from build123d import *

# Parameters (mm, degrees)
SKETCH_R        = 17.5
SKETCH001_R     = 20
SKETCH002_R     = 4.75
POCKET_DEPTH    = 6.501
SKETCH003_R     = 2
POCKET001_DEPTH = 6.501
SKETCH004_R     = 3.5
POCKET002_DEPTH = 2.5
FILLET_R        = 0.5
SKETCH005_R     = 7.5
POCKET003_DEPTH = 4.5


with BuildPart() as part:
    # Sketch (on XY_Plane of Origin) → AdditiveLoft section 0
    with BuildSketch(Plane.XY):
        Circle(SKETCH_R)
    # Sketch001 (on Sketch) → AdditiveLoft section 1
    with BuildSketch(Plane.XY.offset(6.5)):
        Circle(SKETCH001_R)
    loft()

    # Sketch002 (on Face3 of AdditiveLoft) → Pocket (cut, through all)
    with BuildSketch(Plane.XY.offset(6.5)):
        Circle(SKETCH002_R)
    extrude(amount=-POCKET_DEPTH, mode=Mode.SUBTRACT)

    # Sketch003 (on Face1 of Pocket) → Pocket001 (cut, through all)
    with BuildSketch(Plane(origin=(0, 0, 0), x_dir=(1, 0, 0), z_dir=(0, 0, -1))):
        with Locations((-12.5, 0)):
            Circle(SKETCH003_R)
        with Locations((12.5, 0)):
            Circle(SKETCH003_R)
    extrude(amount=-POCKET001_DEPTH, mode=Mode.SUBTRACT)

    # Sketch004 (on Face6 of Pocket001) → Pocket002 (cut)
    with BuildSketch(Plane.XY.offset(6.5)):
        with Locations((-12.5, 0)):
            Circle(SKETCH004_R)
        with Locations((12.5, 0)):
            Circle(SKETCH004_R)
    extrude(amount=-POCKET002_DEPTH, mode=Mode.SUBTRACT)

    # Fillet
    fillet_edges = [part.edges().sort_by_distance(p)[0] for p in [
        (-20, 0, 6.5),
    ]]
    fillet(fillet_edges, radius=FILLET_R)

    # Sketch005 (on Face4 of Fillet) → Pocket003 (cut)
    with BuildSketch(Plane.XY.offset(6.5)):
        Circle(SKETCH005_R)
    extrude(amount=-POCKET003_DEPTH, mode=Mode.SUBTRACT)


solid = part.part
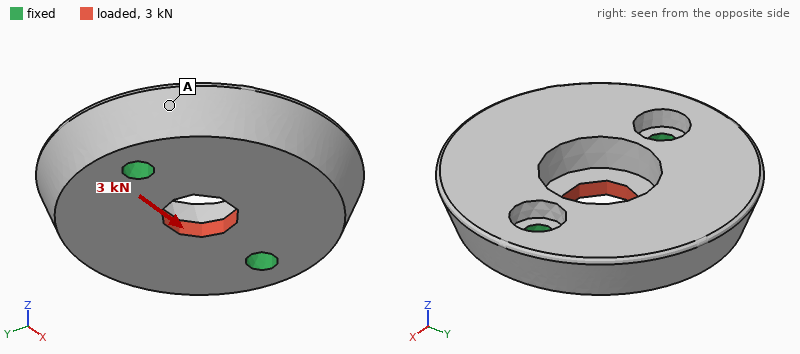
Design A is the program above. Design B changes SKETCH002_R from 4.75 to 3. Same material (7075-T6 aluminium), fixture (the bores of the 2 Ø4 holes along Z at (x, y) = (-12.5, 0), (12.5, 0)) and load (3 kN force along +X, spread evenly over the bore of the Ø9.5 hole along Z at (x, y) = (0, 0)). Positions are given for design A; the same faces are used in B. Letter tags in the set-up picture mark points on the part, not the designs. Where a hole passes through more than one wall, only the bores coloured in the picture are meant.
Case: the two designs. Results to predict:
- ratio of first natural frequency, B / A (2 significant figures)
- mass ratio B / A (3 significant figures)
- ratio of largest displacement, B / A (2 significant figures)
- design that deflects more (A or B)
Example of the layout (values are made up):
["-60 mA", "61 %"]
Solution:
["1.00", "1.01", "1.3", "B"]
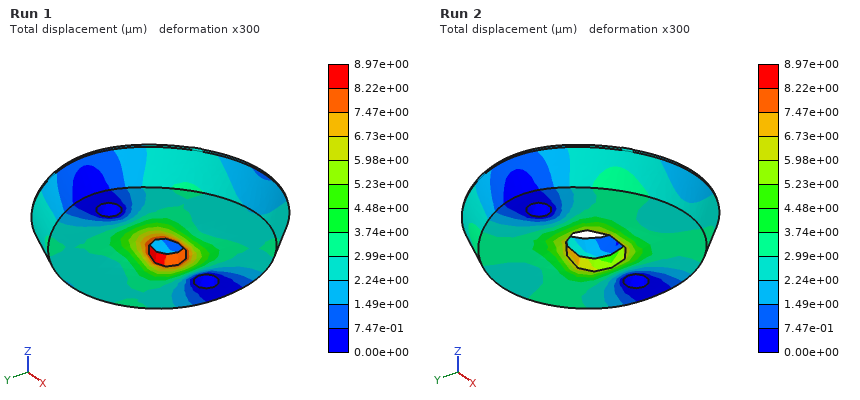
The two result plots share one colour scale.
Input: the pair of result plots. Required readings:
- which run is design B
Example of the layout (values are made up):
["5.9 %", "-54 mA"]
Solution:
["Run 1"]
